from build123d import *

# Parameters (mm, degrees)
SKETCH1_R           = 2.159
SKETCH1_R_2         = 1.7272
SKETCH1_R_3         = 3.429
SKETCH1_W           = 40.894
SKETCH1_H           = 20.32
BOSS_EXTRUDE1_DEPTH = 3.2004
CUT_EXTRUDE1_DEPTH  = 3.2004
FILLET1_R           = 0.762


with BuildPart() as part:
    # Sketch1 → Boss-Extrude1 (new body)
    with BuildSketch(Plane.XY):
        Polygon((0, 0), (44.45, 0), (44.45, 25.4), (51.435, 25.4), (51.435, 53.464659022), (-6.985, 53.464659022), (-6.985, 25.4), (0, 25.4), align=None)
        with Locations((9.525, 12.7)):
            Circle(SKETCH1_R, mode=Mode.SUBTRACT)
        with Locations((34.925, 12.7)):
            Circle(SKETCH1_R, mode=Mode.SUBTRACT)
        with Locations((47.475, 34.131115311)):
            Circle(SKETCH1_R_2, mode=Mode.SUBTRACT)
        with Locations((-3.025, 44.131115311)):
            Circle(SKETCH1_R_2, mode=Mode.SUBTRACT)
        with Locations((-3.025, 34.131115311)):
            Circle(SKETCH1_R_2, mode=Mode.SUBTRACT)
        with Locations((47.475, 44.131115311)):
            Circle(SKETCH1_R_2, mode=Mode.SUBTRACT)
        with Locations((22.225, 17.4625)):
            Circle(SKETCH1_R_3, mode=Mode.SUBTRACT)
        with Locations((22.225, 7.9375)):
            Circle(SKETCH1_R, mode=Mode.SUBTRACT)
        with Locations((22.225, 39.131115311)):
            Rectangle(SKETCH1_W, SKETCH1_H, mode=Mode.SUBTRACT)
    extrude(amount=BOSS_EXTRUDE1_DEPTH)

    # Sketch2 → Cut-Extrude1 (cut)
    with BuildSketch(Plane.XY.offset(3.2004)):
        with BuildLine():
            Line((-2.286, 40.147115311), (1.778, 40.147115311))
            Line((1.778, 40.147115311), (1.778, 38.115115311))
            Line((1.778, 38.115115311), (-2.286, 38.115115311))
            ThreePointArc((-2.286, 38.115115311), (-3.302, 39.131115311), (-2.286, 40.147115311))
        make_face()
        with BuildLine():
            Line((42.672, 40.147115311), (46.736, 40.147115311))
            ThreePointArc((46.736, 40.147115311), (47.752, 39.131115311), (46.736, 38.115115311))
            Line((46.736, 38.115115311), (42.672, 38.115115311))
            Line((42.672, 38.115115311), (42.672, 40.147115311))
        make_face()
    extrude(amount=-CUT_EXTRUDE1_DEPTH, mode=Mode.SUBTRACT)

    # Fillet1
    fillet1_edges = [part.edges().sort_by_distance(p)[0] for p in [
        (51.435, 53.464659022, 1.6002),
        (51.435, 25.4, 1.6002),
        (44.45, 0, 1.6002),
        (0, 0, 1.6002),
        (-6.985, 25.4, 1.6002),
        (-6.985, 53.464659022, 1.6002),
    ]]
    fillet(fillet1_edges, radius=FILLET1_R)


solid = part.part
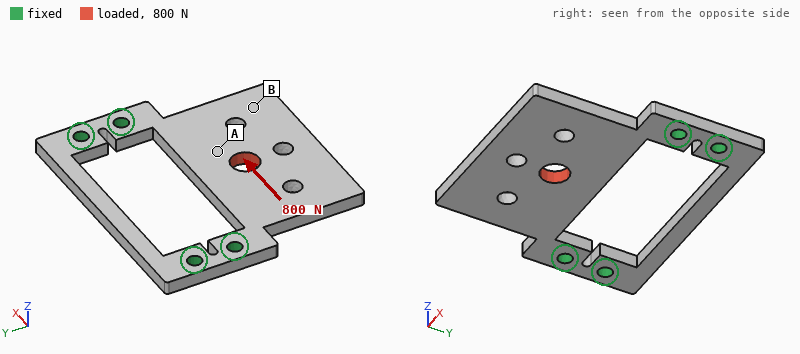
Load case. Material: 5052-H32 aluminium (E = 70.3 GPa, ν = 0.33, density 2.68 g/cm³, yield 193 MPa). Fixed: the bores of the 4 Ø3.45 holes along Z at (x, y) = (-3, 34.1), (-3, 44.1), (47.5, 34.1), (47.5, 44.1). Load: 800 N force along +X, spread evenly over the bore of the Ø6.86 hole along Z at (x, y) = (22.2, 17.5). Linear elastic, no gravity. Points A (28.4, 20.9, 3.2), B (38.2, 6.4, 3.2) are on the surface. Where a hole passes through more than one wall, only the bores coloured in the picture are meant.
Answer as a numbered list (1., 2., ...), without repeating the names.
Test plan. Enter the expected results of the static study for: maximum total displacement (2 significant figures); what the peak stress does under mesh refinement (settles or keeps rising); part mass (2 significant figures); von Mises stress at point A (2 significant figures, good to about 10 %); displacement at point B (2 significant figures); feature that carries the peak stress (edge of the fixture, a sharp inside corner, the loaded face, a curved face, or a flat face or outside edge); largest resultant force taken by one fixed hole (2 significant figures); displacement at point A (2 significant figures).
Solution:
1. 12 µm
2. keeps rising
3. 15 g
4. 11 MPa
5. 11 µm
6. edge of the fixture
7. 460 N
8. 11 µm
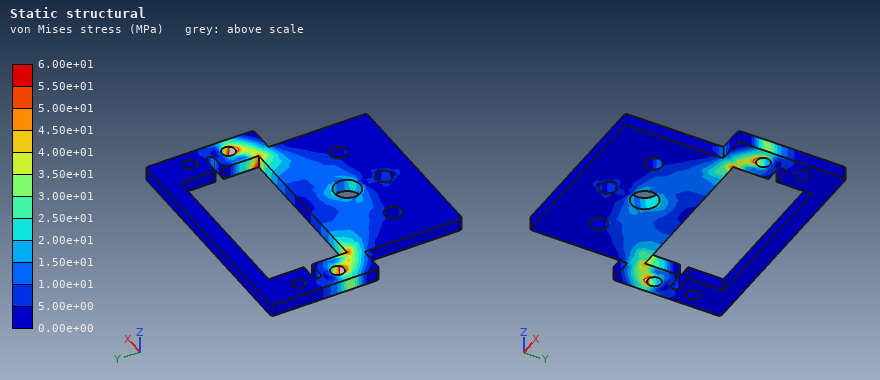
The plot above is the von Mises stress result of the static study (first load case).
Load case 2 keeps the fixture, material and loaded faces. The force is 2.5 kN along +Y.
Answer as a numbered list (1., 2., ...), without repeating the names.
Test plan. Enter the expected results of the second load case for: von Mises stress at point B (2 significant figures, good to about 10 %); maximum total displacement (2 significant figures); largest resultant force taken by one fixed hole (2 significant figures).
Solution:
1. 20 MPa
2. 40 µm
3. 1.4 kN
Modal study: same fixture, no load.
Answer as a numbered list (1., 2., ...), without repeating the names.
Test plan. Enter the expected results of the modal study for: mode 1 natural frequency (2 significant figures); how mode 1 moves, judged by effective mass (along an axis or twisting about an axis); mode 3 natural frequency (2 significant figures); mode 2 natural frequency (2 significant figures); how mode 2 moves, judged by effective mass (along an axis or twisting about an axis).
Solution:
1. 1300 Hz
2. along Z
3. 6000 Hz
4. 4200 Hz
5. twisting about Y
